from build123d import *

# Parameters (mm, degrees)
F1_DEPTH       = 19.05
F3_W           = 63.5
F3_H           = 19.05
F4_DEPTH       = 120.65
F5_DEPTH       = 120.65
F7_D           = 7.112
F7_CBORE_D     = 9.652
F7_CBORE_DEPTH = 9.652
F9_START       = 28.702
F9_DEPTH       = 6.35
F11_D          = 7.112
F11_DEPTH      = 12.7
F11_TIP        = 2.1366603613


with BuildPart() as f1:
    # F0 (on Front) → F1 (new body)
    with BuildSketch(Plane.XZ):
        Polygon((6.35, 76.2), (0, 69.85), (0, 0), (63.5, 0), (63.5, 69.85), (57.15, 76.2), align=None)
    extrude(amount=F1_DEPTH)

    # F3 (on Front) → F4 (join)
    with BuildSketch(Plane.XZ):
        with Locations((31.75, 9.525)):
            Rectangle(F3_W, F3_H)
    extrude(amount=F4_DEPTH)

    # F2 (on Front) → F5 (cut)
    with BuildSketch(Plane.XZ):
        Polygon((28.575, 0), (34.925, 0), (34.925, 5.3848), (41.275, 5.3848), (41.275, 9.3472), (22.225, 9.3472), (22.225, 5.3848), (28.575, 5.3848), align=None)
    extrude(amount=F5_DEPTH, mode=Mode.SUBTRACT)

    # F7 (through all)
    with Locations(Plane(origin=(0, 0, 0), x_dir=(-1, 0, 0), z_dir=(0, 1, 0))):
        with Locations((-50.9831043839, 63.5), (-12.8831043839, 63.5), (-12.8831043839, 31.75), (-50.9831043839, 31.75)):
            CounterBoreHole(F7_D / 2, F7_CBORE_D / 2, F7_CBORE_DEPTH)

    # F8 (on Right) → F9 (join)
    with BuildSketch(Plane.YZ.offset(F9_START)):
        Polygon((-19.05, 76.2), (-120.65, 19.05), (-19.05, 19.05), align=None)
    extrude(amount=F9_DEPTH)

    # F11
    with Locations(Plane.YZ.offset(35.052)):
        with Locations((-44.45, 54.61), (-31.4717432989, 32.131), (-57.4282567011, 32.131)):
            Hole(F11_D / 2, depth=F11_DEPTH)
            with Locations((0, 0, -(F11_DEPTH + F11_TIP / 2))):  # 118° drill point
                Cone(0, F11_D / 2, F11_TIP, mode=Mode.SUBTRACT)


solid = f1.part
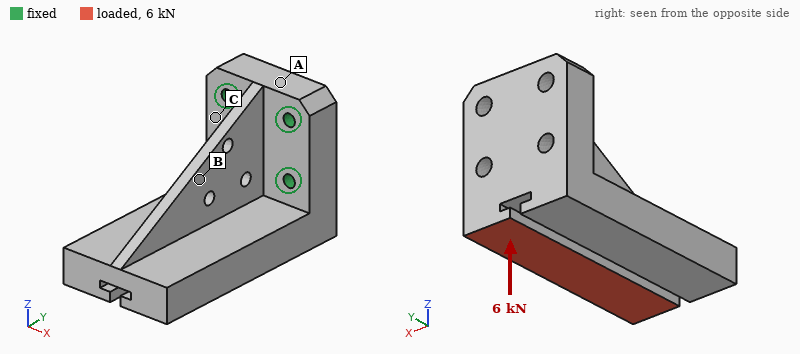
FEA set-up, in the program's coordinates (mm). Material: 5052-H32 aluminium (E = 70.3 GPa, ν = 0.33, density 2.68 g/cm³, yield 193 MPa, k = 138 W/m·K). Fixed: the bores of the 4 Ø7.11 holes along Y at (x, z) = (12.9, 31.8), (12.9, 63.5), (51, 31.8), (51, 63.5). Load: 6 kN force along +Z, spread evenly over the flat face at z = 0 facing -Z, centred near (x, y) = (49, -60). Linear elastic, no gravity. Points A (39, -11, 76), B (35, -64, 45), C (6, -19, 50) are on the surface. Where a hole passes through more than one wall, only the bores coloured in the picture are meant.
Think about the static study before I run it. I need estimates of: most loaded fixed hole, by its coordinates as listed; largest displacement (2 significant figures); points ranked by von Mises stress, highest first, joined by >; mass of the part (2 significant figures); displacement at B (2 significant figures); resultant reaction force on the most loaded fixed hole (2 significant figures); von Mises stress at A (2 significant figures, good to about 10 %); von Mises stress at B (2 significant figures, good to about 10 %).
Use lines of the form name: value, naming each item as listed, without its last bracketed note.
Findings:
most loaded fixed hole, by its coordinates as listed: (51, 31.8)
largest displacement: 0.24 mm
points ranked by von Mises stress, highest first, joined by >: B > A > C
mass of the part: 570 g
displacement at B: 0.076 mm
resultant reaction force on the most loaded fixed hole: 6.0 kN
von Mises stress at A: 21 MPa
von Mises stress at B: 34 MPa
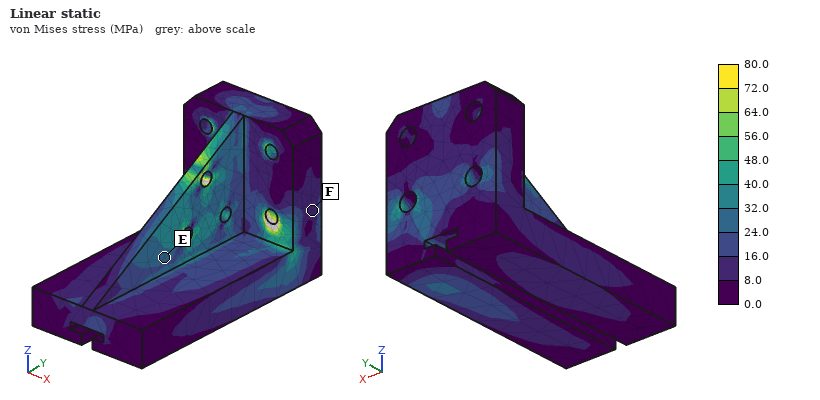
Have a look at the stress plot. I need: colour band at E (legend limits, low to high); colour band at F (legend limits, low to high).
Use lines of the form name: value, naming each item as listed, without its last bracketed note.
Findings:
colour band at E: 24.0 to 32.0 MPa
colour band at F: 8.0 to 16.0 MPa
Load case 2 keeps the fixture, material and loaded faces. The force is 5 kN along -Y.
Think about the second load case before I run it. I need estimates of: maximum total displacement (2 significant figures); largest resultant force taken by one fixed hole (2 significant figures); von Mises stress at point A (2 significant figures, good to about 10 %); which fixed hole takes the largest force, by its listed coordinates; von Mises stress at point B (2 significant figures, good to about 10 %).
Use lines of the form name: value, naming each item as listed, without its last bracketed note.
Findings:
maximum total displacement: 0.12 mm
largest resultant force taken by one fixed hole: 6.4 kN
von Mises stress at point A: 8.5 MPa
which fixed hole takes the largest force, by its listed coordinates: (51, 31.8)
von Mises stress at point B: 11 MPa
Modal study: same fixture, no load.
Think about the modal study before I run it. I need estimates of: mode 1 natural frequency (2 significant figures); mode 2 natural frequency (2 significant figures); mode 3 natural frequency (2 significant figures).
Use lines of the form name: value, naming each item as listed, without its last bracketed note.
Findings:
mode 1 natural frequency: 1800 Hz
mode 2 natural frequency: 1900 Hz
mode 3 natural frequency: 3000 Hz
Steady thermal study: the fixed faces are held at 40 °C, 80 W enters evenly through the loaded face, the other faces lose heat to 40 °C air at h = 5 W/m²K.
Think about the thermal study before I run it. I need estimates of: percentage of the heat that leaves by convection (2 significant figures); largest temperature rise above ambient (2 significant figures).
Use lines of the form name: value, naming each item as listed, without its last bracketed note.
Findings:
percentage of the heat that leaves by convection: 3.7 %
largest temperature rise above ambient: 35 K
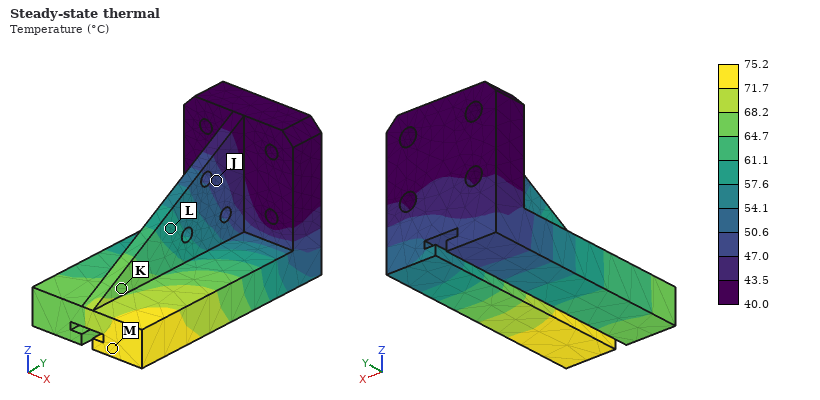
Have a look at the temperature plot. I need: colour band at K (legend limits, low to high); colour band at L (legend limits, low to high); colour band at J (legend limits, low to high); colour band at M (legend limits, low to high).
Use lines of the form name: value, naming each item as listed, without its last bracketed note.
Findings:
colour band at K: 64.7 to 68.2 °C
colour band at L: 57.6 to 61.1 °C
colour band at J: 47.0 to 50.6 °C
colour band at M: 71.7 to 75.2 °C
